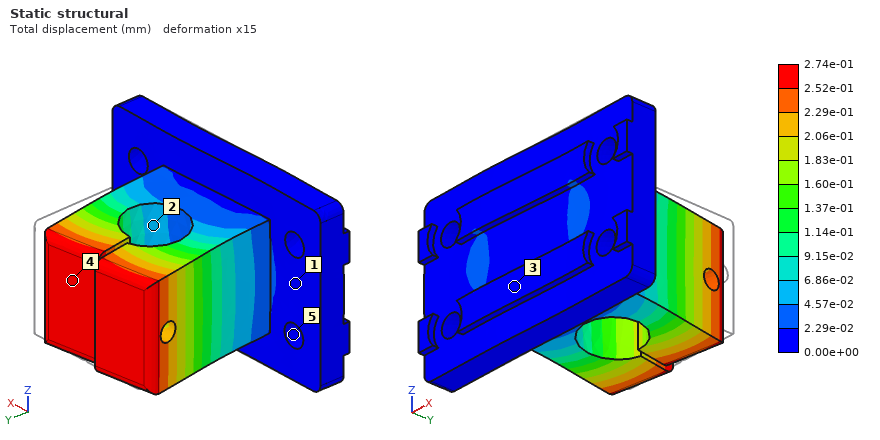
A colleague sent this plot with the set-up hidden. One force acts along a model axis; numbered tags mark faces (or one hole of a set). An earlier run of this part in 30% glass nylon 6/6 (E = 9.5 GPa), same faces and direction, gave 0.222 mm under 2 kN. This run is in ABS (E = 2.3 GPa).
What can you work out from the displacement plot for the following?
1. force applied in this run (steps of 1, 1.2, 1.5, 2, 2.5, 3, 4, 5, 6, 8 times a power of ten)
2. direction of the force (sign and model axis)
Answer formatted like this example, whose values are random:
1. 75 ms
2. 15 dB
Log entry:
1. 600 N
2. -X
